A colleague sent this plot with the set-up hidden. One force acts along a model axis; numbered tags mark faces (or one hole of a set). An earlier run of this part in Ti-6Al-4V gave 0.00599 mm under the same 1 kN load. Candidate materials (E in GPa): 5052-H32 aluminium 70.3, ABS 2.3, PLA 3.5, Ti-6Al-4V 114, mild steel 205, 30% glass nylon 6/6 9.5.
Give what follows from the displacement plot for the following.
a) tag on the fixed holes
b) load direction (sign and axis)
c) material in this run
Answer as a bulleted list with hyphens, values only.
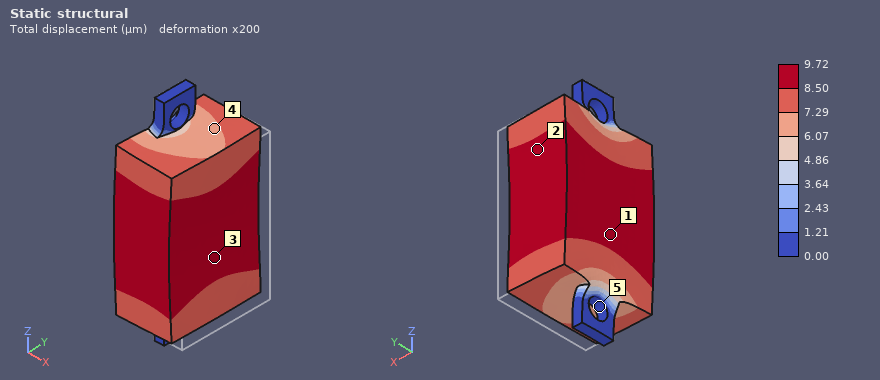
- 5
- -X
- 5052-H32 aluminium
